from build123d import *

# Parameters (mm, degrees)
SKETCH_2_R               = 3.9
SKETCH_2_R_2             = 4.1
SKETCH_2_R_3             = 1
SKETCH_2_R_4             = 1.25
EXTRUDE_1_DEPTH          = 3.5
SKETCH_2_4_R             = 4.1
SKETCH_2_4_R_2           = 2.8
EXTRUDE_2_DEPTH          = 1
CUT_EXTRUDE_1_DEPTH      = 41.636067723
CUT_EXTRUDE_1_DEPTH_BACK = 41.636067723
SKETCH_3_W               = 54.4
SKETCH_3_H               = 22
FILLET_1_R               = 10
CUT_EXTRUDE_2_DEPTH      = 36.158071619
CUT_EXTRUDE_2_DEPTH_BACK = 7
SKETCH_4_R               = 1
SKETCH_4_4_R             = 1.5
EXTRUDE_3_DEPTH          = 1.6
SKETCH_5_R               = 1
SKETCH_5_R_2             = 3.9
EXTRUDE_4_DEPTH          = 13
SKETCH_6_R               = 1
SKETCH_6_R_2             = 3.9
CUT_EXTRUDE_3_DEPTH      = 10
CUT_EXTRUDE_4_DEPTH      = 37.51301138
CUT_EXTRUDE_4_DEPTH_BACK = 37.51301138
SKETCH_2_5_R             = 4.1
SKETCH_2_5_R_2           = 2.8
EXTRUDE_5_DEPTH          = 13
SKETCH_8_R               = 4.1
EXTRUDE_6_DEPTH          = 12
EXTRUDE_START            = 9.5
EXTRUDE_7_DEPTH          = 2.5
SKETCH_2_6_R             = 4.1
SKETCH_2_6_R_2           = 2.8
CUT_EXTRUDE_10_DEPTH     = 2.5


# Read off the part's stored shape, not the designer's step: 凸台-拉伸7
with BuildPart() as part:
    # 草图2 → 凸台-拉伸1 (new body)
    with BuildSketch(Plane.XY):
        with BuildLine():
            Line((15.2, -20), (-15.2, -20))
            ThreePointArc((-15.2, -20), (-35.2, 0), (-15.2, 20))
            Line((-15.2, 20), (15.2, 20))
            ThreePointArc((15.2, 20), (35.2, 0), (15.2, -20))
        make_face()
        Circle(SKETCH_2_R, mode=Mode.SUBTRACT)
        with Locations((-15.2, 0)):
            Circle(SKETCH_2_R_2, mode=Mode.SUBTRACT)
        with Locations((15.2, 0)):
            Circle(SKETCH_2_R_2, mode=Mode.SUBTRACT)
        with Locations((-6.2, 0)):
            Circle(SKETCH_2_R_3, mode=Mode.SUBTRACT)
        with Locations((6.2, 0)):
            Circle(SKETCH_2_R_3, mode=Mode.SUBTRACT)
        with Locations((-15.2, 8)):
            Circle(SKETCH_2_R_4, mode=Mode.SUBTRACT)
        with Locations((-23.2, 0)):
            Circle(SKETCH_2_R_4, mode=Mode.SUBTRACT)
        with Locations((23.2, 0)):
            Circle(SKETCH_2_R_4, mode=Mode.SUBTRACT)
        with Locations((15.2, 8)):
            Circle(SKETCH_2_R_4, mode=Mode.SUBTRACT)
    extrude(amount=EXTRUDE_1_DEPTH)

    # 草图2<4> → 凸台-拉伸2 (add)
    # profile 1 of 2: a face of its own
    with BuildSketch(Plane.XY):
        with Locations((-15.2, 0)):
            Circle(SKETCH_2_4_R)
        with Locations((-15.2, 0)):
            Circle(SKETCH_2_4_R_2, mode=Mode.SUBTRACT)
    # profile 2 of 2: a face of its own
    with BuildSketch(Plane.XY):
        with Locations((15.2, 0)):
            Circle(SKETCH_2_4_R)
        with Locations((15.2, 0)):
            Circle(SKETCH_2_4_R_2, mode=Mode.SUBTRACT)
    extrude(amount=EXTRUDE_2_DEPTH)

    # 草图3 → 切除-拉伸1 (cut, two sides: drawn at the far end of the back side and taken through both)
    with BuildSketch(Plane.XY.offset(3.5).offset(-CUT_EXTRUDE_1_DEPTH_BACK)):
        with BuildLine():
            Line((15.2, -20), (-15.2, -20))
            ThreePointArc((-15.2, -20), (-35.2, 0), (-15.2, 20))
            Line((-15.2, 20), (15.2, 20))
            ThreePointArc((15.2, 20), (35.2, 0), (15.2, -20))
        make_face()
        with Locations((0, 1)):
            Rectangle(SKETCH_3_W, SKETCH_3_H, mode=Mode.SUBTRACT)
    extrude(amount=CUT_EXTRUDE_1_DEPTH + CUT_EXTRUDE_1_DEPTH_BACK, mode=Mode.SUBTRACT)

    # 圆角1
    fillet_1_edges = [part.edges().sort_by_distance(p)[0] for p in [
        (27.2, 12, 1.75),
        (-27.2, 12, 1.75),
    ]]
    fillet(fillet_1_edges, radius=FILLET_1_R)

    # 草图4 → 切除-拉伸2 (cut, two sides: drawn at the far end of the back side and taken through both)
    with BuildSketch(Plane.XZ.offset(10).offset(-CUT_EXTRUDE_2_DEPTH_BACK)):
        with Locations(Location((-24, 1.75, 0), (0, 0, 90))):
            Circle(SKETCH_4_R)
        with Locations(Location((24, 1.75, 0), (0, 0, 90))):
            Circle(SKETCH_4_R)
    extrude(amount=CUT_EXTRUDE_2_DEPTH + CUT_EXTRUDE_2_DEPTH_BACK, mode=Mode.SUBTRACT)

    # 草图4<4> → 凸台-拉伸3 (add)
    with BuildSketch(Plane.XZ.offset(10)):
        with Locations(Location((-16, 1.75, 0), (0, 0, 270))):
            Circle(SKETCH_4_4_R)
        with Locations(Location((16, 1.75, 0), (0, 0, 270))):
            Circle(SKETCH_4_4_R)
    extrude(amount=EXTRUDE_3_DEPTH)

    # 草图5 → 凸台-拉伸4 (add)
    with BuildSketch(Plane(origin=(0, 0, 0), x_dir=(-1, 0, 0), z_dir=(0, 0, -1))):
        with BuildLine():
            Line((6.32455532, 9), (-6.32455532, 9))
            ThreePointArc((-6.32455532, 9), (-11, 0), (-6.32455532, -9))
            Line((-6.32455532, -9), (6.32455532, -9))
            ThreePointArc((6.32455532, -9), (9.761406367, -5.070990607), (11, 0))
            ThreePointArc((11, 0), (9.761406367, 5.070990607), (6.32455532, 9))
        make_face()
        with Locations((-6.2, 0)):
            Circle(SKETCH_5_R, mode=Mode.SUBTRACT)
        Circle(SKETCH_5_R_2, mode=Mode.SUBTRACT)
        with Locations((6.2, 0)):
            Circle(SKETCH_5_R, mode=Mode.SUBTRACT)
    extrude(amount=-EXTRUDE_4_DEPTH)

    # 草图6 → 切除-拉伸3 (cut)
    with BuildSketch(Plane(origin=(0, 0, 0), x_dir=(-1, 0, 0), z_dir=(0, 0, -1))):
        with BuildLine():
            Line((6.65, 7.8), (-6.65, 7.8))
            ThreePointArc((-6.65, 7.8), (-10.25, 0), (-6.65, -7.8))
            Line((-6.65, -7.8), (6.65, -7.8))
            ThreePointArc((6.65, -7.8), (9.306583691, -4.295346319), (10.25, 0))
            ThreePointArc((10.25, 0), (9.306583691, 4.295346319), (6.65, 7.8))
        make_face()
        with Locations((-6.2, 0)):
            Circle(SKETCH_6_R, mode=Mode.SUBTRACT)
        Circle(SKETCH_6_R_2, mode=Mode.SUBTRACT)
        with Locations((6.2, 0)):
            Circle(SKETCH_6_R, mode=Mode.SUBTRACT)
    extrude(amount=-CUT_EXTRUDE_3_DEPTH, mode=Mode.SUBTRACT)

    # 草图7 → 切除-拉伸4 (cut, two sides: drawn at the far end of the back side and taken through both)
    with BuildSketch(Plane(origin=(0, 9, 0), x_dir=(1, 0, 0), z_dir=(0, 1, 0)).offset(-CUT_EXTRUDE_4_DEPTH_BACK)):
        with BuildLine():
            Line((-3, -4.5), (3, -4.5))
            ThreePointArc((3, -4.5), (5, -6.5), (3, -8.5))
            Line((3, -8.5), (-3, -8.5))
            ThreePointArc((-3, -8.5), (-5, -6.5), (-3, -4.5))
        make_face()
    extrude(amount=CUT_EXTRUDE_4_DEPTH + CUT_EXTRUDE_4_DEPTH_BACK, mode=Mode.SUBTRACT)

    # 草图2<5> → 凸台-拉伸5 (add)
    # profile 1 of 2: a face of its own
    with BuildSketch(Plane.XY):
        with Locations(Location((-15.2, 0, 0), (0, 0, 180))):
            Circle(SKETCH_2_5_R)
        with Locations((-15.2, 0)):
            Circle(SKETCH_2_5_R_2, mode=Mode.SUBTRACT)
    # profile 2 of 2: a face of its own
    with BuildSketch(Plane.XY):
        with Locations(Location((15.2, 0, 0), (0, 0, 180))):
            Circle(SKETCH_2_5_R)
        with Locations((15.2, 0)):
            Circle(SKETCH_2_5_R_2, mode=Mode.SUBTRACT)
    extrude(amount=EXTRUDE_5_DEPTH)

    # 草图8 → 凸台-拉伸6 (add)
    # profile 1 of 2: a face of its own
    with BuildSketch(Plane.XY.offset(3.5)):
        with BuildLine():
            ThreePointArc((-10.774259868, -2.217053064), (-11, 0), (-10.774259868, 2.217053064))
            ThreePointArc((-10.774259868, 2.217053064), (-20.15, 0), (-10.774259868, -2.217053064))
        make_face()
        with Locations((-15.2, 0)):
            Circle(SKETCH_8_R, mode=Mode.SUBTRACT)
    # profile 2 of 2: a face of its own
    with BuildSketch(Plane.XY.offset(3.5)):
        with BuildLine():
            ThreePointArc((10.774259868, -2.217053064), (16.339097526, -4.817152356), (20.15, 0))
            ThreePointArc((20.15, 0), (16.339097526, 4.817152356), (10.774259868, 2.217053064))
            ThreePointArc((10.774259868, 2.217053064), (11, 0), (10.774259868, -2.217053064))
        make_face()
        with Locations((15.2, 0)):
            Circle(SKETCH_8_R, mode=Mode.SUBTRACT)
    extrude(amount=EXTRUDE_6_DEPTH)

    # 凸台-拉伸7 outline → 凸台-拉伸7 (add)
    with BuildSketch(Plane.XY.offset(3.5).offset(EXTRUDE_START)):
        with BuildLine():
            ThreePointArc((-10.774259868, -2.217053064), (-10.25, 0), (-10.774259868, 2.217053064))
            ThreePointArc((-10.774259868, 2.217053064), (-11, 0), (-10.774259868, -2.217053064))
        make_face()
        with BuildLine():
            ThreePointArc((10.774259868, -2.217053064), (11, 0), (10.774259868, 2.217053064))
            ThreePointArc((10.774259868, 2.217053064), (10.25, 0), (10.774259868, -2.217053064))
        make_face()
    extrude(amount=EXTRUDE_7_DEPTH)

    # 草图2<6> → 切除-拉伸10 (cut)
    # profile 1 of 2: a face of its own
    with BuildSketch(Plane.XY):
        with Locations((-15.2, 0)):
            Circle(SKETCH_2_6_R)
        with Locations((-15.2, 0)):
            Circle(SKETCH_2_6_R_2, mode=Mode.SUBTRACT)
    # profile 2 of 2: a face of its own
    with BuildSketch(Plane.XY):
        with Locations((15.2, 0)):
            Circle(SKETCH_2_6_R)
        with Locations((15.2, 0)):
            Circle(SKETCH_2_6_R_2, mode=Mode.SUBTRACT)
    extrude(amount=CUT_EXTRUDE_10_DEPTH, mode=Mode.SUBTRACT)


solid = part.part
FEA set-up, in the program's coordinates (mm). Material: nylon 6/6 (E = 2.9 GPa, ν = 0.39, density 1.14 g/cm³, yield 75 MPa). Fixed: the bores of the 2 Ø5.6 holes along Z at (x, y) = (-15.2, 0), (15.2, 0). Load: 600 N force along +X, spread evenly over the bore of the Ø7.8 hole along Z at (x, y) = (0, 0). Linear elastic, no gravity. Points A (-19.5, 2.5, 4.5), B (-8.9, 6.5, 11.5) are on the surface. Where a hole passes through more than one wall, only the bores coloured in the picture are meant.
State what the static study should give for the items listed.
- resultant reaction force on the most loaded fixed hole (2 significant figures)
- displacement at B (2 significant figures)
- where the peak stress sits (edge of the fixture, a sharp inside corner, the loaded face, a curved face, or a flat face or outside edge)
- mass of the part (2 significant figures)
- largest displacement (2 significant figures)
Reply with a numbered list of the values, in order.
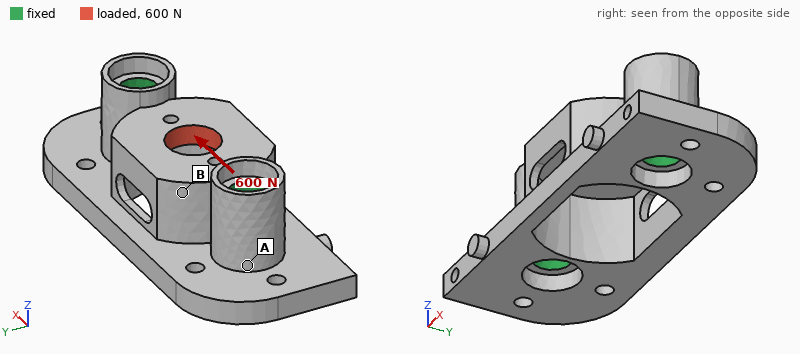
1. 300 N
2. 38 µm
3. a curved face
4. 5.6 g
5. 55 µm
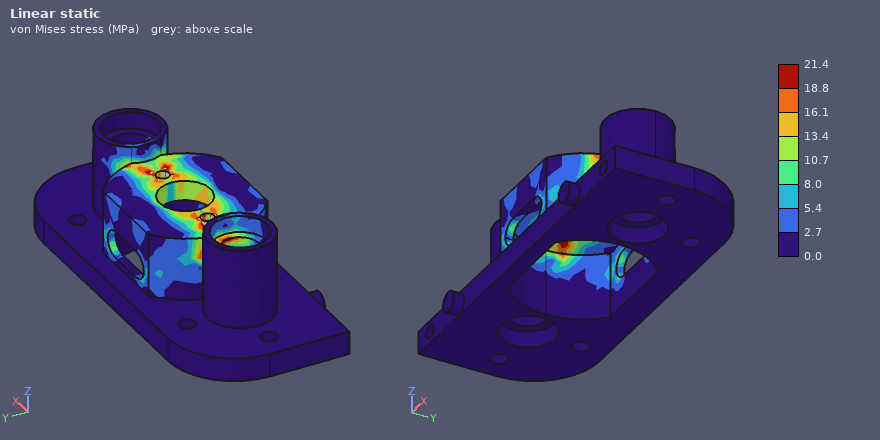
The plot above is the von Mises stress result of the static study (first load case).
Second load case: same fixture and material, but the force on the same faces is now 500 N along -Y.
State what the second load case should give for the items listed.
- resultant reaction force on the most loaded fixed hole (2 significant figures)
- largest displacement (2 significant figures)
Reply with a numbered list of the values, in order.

1. 250 N
2. 0.11 mm
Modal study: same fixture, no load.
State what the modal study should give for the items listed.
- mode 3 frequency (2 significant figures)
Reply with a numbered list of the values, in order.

1. 6500 Hz
